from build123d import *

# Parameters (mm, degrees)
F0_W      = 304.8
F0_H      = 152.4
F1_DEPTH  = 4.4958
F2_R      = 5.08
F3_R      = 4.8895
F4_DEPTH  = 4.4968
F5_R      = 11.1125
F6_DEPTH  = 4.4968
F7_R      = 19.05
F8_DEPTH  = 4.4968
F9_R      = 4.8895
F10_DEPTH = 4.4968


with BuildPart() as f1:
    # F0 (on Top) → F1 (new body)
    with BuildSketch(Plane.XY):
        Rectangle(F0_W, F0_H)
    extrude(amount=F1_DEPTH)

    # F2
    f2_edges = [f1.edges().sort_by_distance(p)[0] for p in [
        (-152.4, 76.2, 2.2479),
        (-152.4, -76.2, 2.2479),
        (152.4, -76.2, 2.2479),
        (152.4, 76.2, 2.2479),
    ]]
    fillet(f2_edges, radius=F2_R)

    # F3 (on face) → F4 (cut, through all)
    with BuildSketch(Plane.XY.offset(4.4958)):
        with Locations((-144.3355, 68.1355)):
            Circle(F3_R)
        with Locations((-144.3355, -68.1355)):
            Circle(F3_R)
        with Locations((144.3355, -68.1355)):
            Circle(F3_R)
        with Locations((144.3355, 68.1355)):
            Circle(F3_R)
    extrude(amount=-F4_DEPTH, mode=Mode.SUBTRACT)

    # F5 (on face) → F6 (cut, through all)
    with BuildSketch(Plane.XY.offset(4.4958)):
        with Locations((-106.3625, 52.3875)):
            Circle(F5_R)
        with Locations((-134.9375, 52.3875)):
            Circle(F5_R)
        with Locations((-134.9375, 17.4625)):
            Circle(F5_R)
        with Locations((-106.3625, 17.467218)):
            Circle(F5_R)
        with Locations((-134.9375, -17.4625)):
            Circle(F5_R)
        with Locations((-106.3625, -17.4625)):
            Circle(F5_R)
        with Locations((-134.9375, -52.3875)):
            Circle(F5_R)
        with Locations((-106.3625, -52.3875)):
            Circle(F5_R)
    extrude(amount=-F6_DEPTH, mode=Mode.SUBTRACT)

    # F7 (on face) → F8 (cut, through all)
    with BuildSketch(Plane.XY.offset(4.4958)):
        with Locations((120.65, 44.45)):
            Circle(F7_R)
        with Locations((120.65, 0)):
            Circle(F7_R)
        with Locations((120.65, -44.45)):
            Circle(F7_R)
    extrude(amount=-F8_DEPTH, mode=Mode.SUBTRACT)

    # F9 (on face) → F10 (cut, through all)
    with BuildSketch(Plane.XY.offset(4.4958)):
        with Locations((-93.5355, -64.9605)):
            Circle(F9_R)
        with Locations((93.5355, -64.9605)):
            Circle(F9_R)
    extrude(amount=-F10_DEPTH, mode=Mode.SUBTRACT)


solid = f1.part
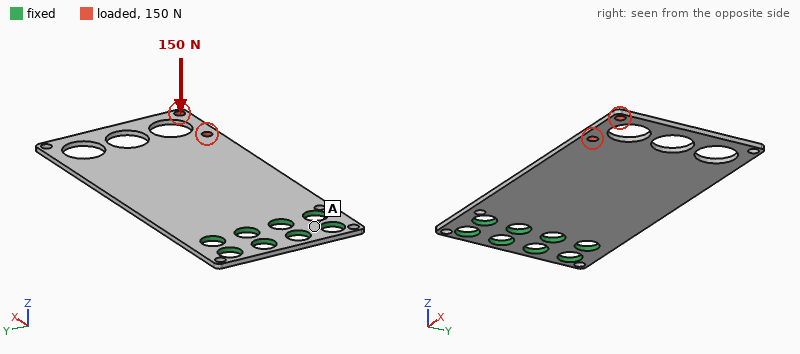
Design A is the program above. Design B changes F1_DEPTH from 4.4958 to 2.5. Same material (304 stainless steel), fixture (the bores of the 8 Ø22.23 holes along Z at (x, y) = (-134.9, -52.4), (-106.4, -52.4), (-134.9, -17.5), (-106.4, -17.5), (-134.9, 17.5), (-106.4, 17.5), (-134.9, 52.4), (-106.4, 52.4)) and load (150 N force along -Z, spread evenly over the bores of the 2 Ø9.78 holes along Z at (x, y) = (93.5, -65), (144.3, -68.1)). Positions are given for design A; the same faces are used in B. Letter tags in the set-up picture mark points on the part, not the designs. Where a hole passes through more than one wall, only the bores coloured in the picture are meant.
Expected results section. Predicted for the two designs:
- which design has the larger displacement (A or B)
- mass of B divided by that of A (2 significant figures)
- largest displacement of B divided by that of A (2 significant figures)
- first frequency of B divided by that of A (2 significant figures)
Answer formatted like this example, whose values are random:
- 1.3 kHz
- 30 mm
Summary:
- B
- 0.56
- 5.8
- 0.56
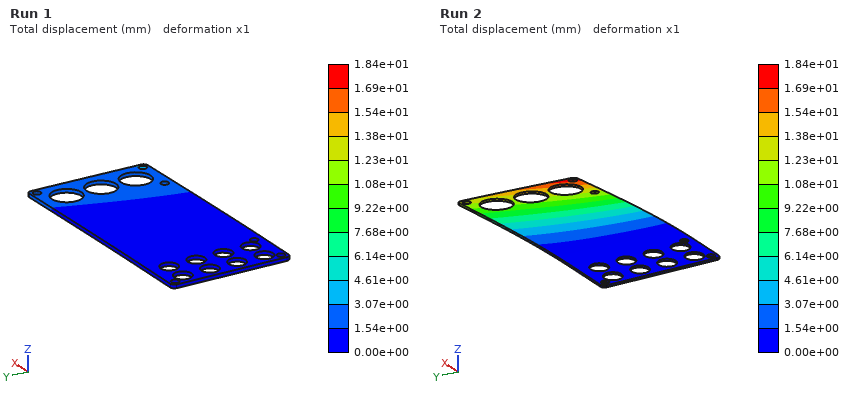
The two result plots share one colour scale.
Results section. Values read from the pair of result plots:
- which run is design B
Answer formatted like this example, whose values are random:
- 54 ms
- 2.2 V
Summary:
- Run 2
